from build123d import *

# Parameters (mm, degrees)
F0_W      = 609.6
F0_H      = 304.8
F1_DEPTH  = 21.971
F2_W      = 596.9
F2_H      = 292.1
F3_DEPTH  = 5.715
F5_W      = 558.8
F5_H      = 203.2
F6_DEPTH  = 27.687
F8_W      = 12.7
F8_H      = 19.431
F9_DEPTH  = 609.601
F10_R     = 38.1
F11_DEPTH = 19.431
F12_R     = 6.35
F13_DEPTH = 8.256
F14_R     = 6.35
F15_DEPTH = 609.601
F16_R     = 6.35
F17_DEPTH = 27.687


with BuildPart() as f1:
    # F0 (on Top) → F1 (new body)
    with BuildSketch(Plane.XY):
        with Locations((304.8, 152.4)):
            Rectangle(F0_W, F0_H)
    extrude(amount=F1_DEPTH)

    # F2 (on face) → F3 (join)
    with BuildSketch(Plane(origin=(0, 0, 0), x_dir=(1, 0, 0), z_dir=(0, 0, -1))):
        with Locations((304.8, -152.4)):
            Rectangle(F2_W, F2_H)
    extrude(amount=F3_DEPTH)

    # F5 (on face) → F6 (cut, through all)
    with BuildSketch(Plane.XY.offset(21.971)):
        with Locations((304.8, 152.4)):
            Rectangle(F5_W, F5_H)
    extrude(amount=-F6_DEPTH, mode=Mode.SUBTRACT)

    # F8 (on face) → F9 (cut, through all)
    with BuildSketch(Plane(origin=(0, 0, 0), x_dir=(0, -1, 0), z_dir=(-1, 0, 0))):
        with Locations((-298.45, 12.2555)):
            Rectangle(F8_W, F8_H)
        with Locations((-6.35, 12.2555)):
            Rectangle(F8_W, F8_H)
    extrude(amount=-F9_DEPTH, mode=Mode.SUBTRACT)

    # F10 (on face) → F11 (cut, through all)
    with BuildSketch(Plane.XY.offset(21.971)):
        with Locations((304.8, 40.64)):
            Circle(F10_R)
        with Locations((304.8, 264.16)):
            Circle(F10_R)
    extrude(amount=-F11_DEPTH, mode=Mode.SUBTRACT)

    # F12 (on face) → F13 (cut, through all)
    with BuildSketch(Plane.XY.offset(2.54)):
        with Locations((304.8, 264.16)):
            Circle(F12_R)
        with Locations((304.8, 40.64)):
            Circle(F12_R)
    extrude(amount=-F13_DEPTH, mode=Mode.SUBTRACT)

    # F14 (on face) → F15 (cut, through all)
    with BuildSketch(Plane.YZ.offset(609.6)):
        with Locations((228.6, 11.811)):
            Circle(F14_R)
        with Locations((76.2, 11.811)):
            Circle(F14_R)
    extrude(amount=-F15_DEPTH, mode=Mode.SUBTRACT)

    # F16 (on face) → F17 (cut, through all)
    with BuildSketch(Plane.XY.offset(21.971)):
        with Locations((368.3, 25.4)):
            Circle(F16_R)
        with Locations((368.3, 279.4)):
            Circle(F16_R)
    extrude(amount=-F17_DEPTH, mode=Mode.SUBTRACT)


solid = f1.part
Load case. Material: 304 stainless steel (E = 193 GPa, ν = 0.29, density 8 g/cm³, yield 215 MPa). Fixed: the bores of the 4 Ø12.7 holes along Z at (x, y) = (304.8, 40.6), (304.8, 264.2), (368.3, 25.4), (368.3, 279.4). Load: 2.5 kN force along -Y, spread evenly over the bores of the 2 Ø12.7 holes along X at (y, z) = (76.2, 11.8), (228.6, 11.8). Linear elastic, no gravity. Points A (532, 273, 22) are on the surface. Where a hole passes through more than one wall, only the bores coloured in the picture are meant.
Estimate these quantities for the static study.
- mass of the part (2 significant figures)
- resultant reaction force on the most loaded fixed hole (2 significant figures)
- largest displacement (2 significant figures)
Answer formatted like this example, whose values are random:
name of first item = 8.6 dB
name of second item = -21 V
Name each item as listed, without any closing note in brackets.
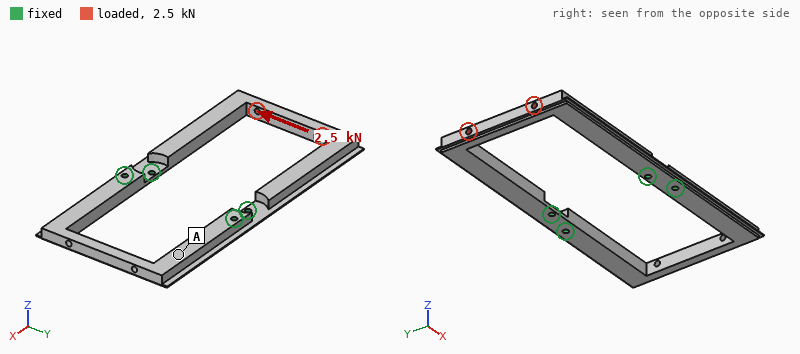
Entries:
mass of the part = 12 kg
resultant reaction force on the most loaded fixed hole = 4.4 kN
largest displacement = 0.32 mm
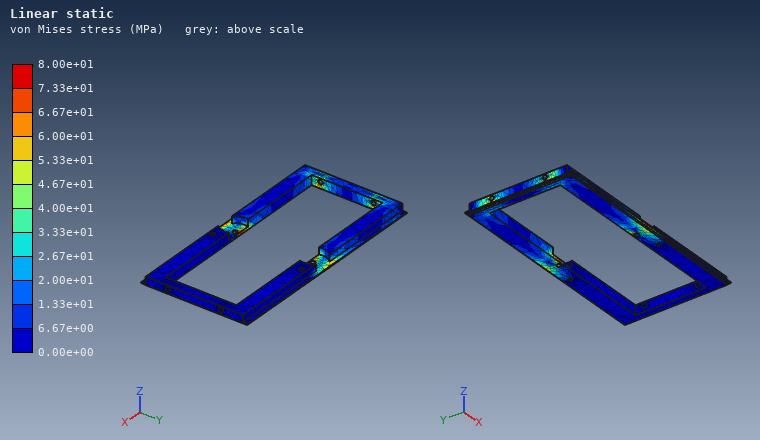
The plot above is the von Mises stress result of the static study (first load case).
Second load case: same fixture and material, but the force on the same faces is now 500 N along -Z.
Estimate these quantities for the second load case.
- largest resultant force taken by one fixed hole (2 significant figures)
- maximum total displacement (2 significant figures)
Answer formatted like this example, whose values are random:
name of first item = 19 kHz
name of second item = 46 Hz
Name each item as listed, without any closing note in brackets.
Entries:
largest resultant force taken by one fixed hole = 830 N
maximum total displacement = 1.7 mm
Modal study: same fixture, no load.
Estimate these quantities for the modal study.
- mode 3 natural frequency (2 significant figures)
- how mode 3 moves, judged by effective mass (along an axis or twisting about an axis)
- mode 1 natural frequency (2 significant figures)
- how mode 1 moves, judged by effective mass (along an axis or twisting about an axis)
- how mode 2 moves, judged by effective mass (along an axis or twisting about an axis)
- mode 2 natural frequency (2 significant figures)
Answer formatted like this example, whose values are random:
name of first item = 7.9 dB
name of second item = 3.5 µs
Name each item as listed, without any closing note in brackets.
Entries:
mode 3 natural frequency = 270 Hz
how mode 3 moves, judged by effective mass = along Y
mode 1 natural frequency = 53 Hz
how mode 1 moves, judged by effective mass = along Z
how mode 2 moves, judged by effective mass = twisting about X
mode 2 natural frequency = 170 Hz
